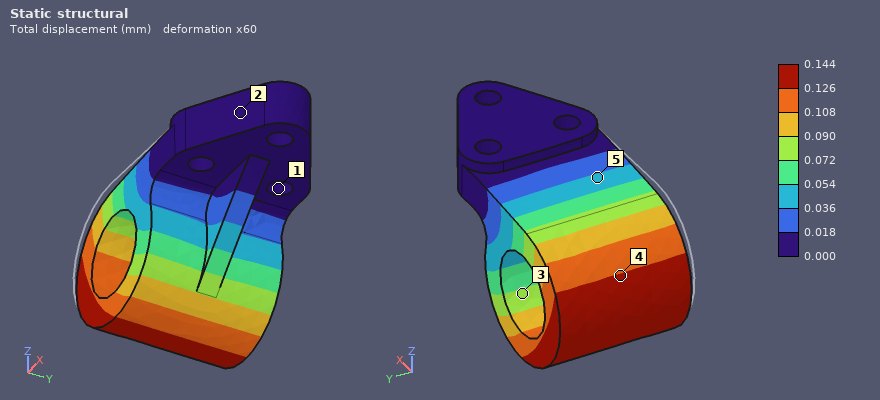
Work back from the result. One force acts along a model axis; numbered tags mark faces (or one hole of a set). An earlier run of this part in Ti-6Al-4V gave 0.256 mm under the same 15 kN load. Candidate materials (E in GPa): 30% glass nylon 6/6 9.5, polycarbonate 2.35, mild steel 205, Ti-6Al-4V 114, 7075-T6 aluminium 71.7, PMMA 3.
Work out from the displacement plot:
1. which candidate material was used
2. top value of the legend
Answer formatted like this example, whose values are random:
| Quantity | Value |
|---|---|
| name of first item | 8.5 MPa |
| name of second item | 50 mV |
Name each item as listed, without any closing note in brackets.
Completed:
| Quantity | Value |
|---|---|
| which candidate material was used | mild steel |
| top value of the legend | 0.144 mm |
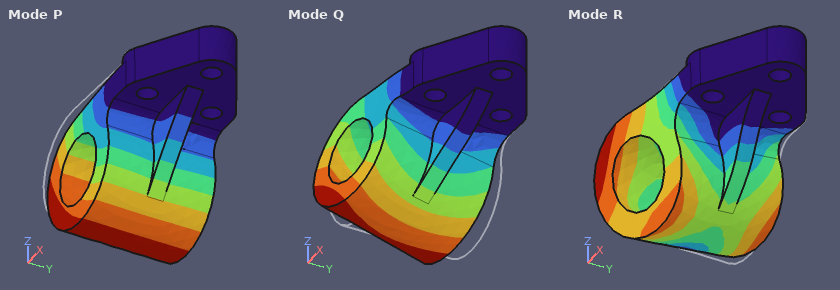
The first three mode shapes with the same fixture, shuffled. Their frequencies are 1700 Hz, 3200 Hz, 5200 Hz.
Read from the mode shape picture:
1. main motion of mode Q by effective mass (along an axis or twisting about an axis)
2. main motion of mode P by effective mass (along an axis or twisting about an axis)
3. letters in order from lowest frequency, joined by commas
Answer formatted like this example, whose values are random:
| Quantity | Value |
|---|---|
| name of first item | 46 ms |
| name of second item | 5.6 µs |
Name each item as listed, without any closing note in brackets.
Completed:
| Quantity | Value |
|---|---|
| main motion of mode Q by effective mass | along Y |
| main motion of mode P by effective mass | along Z |
| letters in order from lowest frequency, joined by commas | P, Q, R |
